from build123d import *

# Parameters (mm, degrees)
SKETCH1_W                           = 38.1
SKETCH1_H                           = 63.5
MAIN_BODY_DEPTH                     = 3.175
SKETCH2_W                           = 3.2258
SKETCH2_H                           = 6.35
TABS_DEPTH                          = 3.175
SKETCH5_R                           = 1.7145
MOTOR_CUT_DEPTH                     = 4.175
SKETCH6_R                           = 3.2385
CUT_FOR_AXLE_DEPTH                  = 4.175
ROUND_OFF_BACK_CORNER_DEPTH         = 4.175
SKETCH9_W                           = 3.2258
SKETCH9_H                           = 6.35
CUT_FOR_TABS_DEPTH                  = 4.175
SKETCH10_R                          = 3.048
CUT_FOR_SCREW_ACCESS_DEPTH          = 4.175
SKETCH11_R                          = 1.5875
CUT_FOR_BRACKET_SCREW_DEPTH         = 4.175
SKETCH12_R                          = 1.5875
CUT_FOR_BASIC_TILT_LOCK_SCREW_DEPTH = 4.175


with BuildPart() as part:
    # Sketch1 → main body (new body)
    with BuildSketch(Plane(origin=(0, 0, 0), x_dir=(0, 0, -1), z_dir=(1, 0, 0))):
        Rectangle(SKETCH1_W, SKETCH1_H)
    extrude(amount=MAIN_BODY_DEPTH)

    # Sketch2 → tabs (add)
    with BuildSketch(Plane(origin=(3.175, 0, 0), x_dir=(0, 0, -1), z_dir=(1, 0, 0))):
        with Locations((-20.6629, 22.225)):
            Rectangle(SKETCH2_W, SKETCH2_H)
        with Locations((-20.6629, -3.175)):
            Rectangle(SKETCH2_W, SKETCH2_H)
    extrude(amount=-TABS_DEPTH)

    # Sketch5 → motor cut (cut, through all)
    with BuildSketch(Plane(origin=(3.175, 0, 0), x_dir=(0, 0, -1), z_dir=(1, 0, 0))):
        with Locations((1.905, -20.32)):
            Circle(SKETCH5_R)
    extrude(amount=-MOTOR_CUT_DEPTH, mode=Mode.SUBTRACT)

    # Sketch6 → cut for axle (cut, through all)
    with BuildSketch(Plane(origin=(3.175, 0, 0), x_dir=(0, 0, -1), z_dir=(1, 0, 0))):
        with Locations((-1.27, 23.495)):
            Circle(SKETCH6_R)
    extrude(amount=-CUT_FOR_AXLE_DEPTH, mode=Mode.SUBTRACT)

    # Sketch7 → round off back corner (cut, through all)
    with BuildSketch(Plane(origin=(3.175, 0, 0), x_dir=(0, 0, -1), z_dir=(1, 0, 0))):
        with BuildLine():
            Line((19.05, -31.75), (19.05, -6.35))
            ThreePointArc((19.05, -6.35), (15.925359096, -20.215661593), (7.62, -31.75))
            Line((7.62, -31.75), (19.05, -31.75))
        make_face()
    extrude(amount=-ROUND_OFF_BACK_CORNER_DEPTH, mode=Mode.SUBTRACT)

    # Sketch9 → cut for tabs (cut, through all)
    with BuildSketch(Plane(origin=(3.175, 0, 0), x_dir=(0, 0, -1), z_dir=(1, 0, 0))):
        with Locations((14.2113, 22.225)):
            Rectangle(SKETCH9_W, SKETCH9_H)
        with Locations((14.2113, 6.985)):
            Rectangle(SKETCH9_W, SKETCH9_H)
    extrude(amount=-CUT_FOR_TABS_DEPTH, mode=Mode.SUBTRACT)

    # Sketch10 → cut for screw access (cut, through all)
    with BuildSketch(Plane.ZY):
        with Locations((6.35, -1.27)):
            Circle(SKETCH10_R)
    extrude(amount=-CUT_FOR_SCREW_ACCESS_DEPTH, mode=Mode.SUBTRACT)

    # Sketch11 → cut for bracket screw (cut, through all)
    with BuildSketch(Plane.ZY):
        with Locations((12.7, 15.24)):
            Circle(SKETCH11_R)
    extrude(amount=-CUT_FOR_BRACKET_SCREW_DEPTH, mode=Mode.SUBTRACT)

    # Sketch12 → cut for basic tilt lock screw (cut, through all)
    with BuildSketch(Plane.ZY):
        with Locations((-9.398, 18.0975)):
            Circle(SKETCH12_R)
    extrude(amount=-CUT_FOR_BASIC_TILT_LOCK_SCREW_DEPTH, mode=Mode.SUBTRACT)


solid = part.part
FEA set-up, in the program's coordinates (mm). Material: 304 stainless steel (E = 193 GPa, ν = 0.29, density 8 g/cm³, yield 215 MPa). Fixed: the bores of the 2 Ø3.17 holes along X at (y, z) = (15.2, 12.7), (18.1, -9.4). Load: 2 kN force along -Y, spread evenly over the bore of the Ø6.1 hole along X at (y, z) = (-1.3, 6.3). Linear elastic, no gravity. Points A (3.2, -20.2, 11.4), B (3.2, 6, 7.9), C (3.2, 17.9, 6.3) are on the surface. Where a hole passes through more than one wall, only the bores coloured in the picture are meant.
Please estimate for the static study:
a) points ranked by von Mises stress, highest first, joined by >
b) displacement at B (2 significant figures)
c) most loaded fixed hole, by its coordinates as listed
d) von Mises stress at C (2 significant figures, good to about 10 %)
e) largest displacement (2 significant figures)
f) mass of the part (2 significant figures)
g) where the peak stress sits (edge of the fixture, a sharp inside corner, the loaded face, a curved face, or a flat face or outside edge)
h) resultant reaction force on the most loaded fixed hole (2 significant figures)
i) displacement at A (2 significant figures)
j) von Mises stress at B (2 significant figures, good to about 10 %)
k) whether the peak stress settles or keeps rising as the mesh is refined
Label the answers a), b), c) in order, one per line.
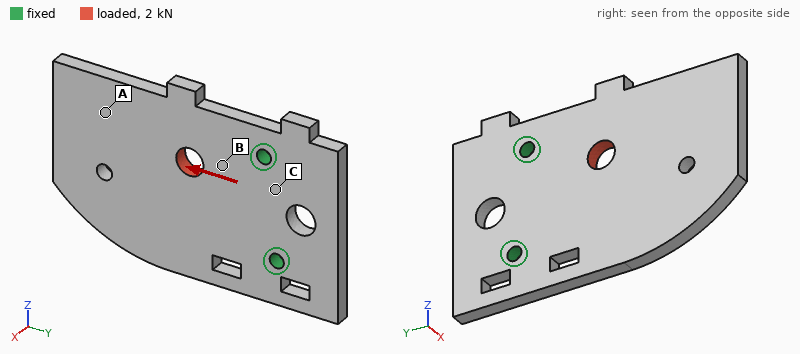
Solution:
a) B > C > A
b) 1.9 µm
c) (15.2, 12.7)
d) 12 MPa
e) 4.4 µm
f) 57 g
g) edge of the fixture
h) 1.4 kN
i) 3.4 µm
j) 33 MPa
k) keeps rising
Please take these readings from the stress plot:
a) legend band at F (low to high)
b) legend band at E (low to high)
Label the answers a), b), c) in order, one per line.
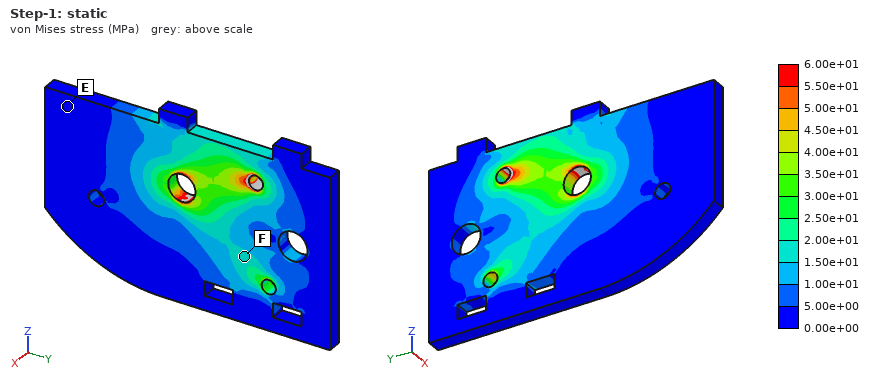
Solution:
a) 1.50e+01 to 2.00e+01 MPa
b) 0.00e+00 to 5.00e+00 MPa
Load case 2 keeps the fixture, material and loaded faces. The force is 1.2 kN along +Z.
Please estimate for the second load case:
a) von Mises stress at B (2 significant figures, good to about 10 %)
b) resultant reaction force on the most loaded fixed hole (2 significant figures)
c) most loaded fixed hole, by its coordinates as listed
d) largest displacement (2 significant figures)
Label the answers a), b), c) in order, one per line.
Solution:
a) 31 MPa
b) 1.1 kN
c) (15.2, 12.7)
d) 8.8 µm
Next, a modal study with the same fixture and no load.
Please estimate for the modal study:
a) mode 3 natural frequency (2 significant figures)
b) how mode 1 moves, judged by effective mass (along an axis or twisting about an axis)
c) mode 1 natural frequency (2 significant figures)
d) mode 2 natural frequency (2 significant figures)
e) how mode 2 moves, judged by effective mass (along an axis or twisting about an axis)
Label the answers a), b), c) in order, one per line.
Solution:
a) 6500 Hz
b) along X
c) 1100 Hz
d) 3400 Hz
e) twisting about Y
